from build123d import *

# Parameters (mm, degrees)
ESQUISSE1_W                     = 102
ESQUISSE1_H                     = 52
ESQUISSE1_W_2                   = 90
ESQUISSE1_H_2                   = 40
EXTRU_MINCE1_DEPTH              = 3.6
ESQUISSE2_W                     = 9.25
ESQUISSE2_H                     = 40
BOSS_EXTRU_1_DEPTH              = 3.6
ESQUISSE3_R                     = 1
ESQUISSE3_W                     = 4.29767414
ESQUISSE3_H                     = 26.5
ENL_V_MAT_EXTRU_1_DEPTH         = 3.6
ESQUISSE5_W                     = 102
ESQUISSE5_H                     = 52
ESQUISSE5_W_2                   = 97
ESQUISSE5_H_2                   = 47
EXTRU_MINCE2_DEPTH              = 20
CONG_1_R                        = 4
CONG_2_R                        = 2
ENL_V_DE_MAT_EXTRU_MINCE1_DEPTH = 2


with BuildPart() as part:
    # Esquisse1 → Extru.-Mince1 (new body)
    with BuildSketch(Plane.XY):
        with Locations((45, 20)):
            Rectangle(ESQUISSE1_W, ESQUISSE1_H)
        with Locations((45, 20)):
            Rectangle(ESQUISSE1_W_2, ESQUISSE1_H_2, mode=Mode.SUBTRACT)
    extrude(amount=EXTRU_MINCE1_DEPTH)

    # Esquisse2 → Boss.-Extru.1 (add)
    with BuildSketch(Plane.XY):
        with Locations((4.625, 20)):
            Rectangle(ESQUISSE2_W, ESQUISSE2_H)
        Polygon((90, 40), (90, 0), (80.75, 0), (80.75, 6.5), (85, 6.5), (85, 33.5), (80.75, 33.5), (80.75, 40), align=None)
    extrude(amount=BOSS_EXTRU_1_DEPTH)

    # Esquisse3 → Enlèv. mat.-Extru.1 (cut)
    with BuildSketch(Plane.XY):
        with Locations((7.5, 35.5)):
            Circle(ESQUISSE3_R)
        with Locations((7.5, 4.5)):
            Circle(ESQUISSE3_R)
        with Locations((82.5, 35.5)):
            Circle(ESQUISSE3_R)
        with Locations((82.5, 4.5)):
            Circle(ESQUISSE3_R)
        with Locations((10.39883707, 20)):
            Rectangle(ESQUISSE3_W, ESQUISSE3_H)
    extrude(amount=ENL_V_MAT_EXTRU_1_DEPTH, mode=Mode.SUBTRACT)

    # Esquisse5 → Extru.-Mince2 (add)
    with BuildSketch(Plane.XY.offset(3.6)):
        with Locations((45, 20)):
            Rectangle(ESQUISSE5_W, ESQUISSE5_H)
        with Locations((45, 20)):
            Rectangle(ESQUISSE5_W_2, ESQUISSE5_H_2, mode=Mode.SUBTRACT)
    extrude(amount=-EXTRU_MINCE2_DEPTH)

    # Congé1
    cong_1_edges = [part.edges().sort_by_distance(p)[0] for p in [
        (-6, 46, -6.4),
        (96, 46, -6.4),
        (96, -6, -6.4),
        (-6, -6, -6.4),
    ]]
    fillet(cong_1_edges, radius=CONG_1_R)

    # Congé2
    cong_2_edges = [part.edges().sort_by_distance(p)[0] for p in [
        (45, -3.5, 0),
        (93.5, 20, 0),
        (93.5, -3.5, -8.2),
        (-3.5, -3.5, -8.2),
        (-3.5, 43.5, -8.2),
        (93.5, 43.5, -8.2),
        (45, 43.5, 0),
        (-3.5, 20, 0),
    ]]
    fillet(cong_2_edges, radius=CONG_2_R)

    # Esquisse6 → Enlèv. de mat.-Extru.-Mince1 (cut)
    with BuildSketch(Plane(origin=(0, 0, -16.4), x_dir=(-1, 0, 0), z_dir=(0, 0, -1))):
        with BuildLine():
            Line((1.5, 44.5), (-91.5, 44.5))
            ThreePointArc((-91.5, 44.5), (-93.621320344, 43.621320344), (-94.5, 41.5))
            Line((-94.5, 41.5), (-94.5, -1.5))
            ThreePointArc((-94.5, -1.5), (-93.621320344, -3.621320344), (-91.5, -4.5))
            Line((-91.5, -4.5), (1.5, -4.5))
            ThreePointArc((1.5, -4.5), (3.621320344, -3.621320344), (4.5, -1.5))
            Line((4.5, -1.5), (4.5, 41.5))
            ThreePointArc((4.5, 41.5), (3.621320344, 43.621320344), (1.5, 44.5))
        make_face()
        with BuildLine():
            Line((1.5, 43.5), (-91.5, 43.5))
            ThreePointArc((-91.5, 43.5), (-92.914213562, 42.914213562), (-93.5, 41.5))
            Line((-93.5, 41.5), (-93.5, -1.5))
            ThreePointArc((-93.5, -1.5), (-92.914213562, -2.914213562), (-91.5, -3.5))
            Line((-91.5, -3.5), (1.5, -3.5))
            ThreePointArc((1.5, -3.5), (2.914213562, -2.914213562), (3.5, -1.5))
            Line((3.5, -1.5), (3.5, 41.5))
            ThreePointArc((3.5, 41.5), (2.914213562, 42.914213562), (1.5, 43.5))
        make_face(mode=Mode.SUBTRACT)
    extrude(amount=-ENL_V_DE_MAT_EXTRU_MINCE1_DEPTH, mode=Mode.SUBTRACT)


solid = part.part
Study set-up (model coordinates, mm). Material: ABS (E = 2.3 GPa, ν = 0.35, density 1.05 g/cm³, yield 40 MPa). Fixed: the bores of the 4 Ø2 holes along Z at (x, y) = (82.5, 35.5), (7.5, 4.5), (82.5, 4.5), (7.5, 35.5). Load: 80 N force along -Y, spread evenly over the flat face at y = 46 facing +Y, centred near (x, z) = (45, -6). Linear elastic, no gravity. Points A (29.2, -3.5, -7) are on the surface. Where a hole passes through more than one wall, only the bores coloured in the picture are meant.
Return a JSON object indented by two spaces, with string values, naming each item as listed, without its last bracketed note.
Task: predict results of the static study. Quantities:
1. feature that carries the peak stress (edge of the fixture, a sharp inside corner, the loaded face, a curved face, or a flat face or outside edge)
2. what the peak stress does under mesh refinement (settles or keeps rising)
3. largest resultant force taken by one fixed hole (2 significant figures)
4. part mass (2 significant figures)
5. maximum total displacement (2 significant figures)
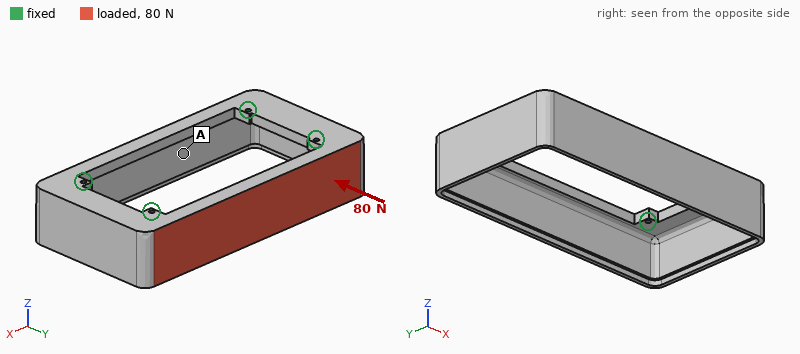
{
  "feature that carries the peak stress": "a sharp inside corner",
  "what the peak stress does under mesh refinement": "keeps rising",
  "largest resultant force taken by one fixed hole": "55 N",
  "part mass": "21 g",
  "maximum total displacement": "1.2 mm"
}
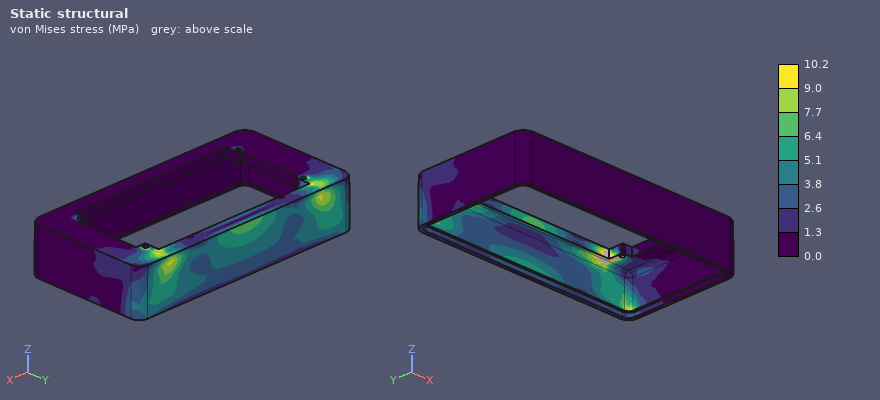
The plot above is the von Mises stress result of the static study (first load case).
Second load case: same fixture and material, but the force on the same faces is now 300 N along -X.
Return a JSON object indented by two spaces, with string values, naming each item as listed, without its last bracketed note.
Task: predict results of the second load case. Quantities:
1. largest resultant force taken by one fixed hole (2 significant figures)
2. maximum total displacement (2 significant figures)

{
  "largest resultant force taken by one fixed hole": "190 N",
  "maximum total displacement": "0.19 mm"
}
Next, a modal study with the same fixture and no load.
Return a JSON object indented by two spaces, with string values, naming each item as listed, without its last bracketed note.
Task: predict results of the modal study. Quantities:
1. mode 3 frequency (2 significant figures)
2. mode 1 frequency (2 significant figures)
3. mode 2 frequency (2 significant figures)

{
  "mode 3 frequency": "1600 Hz",
  "mode 1 frequency": "780 Hz",
  "mode 2 frequency": "800 Hz"
}
